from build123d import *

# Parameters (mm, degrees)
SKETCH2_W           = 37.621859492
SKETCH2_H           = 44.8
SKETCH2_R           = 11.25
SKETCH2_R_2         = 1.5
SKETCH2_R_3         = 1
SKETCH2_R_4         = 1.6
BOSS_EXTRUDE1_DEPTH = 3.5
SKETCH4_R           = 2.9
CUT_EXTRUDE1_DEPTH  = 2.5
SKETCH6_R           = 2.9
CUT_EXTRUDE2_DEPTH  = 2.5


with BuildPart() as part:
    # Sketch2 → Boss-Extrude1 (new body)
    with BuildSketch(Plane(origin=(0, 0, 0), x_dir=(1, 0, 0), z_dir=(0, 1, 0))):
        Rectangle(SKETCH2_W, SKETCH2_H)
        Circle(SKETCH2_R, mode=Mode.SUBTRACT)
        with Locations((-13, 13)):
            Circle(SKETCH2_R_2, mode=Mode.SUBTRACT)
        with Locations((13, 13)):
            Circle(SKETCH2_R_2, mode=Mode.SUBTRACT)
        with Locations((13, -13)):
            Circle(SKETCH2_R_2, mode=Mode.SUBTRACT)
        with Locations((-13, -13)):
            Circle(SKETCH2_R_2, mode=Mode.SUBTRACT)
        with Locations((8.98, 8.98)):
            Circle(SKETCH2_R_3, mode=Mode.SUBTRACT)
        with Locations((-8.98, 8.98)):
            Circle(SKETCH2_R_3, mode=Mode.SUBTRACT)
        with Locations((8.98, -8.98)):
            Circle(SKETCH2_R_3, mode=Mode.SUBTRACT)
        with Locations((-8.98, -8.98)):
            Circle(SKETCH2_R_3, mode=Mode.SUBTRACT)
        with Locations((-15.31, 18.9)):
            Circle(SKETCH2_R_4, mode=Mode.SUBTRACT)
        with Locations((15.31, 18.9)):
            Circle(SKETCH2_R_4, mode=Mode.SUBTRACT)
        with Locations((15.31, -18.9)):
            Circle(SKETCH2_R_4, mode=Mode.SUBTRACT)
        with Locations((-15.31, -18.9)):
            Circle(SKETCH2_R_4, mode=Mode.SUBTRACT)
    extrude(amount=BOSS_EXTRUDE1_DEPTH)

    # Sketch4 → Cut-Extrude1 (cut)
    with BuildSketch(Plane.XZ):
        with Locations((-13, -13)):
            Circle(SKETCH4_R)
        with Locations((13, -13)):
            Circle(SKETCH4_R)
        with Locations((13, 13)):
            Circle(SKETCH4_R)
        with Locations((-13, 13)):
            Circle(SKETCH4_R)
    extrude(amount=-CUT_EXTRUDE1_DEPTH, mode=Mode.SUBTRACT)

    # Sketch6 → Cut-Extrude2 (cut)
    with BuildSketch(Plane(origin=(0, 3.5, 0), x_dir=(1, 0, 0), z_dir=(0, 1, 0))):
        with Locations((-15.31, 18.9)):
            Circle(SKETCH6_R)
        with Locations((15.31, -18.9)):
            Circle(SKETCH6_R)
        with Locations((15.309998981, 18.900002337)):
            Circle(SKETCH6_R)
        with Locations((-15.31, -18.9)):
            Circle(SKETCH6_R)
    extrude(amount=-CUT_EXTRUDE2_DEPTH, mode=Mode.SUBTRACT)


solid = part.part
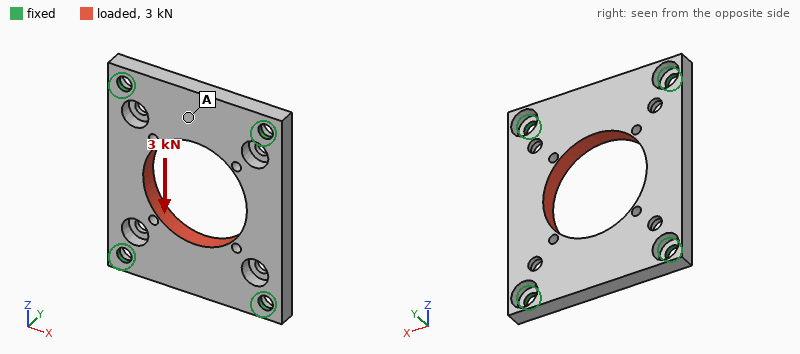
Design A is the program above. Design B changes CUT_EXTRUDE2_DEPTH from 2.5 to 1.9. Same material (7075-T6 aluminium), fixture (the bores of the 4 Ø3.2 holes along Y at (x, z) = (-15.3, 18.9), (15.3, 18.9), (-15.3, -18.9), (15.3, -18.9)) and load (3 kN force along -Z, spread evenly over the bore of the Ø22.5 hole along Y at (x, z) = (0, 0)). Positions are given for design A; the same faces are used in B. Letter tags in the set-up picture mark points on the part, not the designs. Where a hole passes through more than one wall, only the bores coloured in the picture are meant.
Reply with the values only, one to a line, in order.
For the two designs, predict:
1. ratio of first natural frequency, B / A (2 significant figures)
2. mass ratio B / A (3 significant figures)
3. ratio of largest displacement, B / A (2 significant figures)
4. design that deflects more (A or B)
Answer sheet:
1.1
1.01
0.75
A
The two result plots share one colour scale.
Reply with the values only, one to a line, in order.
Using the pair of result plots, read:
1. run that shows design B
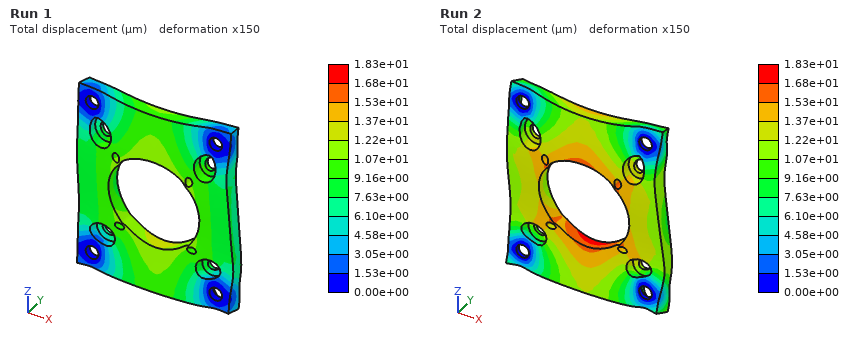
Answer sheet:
Run 1
